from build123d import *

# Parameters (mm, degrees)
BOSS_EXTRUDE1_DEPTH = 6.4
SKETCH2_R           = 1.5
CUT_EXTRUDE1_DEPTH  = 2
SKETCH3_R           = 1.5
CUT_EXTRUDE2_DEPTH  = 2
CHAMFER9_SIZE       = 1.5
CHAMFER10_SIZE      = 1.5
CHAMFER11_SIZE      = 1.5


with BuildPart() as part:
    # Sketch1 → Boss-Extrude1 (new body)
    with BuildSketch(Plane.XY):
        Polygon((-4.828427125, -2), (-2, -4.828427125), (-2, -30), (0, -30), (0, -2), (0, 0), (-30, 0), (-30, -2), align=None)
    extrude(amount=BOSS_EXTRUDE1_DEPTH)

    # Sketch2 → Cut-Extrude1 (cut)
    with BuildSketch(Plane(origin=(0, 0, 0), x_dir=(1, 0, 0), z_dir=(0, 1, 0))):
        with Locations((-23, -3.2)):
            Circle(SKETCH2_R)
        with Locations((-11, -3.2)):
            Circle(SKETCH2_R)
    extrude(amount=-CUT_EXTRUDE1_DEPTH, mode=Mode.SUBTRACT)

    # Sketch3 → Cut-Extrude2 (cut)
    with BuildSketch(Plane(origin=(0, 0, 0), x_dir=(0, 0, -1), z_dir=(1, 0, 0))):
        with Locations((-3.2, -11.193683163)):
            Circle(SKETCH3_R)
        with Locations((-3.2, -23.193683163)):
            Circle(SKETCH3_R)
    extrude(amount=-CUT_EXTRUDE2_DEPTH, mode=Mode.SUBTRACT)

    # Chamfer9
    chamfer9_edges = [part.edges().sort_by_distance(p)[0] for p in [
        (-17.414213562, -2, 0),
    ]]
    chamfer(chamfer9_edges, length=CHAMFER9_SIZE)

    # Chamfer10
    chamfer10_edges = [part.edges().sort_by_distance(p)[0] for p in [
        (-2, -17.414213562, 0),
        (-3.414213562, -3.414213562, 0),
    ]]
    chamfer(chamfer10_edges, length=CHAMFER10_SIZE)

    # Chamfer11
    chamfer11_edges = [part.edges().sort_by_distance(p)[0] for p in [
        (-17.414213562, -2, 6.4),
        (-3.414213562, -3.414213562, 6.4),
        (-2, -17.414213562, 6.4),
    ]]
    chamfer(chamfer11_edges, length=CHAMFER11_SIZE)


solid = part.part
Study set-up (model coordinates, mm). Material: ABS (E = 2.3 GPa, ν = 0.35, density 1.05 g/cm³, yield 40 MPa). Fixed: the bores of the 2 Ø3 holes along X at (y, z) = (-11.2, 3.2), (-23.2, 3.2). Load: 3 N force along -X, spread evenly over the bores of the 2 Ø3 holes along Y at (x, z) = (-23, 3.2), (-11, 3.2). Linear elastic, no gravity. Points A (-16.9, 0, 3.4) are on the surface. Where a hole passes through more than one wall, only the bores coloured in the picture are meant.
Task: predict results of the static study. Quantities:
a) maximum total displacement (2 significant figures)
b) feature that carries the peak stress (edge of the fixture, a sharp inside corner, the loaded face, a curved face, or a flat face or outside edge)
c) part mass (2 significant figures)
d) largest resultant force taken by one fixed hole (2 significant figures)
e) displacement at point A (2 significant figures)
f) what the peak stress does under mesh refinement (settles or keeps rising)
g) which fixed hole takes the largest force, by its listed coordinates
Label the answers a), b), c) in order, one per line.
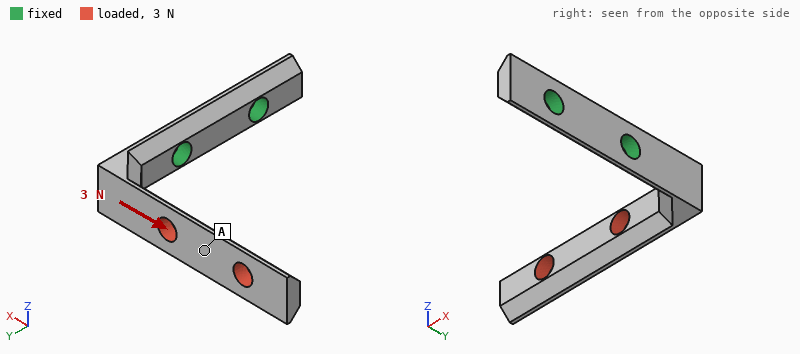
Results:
a) 0.42 mm
b) edge of the fixture
c) 0.62 g
d) 3.0 N
e) 0.25 mm
f) keeps rising
g) (-11.2, 3.2)
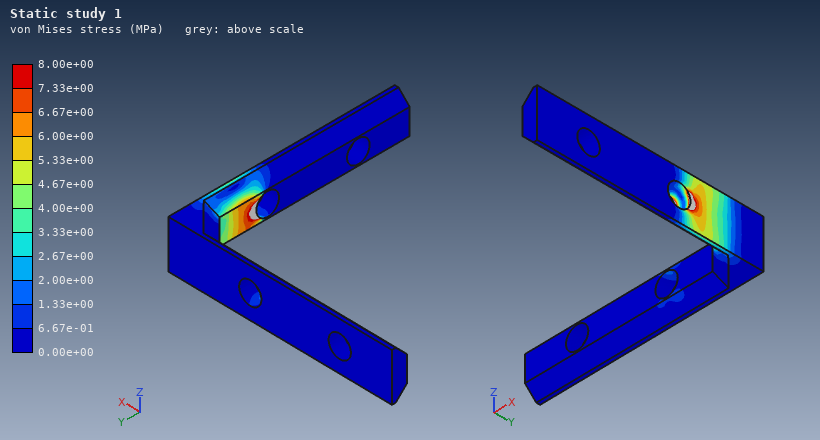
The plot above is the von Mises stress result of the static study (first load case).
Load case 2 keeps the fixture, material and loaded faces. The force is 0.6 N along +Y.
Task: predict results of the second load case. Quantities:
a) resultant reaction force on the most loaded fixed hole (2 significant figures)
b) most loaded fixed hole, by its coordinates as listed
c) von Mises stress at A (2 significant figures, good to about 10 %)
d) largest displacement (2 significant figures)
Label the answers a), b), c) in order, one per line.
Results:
a) 0.70 N
b) (-11.2, 3.2)
c) 0.51 MPa
d) 0.46 mm
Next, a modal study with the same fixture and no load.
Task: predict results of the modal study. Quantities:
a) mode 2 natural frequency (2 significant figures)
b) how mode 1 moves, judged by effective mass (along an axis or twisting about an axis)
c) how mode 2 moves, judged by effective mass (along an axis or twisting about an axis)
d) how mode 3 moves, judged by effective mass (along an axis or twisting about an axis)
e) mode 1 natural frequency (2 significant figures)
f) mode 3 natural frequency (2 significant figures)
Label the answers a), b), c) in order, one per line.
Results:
a) 640 Hz
b) along Y
c) along Z
d) along X
e) 430 Hz
f) 1700 Hz
